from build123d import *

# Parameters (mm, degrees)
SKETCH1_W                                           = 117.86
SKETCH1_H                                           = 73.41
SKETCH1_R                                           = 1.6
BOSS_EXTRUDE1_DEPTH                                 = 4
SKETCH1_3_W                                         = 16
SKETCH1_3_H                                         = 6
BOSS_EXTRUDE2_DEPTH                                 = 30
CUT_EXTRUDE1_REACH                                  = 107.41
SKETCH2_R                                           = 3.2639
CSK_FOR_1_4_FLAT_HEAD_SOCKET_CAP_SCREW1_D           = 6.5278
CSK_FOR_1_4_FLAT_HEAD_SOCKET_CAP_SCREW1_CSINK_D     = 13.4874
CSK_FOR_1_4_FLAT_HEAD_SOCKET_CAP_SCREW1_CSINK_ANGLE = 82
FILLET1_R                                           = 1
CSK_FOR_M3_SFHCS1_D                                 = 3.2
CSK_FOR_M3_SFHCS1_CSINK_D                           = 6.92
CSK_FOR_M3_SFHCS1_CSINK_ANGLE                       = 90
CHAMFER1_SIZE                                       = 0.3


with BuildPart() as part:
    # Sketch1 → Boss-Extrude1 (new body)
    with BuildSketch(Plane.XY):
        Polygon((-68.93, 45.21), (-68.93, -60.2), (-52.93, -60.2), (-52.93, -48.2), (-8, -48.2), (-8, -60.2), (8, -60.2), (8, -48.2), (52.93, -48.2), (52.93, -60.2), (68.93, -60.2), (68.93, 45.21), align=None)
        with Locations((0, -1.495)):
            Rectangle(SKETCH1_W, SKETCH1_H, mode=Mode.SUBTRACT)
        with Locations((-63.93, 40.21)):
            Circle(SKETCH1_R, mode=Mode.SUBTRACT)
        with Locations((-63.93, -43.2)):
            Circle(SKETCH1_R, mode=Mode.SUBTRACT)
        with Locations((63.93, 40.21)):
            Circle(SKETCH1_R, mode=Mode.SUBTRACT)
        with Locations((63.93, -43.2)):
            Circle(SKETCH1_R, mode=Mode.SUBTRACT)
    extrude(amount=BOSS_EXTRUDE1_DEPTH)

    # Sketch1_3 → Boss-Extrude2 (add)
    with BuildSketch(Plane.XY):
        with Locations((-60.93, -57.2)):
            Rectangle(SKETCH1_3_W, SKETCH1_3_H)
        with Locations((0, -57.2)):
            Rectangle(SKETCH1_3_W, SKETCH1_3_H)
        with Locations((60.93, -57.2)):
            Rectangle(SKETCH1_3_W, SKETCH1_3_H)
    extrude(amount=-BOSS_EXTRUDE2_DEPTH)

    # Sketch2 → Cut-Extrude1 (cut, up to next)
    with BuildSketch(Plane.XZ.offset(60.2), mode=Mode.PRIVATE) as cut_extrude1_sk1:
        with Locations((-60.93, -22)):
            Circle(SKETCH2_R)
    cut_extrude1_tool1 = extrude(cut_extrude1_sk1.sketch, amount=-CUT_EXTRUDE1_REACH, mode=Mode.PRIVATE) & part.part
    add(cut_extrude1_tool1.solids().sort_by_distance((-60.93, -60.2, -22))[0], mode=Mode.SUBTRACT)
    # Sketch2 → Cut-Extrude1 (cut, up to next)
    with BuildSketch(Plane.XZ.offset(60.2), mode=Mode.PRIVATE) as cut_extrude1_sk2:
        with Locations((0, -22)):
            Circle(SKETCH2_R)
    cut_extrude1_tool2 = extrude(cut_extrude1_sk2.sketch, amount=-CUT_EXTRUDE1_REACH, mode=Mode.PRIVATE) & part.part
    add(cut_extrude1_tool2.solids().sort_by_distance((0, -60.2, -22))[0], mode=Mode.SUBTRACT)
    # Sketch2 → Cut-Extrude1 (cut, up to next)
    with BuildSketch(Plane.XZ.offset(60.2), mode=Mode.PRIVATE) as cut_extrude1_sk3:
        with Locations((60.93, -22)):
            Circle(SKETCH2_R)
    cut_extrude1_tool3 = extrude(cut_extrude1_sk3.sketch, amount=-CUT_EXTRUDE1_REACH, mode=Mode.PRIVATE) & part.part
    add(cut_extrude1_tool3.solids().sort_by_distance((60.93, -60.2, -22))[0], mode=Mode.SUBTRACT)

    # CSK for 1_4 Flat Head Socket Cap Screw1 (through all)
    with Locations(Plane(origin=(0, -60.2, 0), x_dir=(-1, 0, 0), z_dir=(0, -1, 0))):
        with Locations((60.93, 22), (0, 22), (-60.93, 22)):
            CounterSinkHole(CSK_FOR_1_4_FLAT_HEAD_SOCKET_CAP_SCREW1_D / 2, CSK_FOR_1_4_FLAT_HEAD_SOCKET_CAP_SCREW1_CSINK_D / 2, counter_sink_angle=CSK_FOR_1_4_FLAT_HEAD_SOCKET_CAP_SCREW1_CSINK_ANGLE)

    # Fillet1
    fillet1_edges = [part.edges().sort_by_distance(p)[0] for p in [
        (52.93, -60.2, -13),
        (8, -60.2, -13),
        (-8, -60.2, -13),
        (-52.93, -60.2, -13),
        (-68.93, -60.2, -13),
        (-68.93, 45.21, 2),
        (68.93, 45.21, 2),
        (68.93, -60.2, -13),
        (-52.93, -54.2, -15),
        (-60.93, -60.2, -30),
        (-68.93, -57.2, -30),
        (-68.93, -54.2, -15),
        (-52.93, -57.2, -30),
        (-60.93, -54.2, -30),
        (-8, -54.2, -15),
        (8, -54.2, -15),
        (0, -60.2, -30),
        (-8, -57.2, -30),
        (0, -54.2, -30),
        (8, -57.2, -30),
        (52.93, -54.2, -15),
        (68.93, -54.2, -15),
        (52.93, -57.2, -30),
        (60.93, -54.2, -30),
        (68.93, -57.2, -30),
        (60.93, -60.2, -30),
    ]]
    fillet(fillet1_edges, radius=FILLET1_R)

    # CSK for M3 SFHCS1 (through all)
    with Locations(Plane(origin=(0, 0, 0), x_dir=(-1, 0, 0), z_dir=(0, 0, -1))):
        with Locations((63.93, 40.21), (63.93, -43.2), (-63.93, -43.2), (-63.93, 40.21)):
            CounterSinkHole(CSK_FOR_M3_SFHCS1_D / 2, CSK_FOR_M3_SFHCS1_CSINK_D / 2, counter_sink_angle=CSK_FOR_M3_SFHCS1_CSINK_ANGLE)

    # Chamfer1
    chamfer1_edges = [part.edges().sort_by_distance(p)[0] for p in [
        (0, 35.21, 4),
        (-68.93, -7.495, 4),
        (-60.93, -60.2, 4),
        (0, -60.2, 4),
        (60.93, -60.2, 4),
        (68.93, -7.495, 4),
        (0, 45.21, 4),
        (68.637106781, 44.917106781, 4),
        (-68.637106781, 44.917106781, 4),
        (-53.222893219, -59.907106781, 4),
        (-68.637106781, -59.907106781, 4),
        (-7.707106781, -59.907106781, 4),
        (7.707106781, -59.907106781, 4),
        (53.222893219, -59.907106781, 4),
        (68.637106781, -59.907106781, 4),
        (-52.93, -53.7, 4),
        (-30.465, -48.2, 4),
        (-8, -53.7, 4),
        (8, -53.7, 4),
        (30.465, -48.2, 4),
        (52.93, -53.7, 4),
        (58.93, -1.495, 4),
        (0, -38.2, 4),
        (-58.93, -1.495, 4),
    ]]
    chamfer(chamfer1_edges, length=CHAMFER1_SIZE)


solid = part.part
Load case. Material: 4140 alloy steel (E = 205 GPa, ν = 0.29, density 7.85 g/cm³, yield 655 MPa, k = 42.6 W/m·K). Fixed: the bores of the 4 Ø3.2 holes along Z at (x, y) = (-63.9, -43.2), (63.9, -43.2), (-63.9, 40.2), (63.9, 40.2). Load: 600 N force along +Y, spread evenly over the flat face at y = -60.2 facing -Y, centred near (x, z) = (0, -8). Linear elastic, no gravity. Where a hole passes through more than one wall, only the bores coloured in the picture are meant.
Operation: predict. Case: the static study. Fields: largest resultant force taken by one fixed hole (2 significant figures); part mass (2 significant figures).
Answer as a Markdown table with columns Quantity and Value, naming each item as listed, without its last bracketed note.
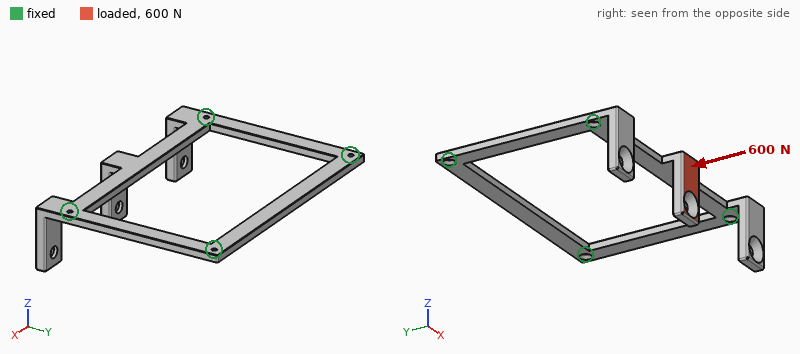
| Quantity | Value |
|---|---|
| largest resultant force taken by one fixed hole | 210 N |
| part mass | 210 g |
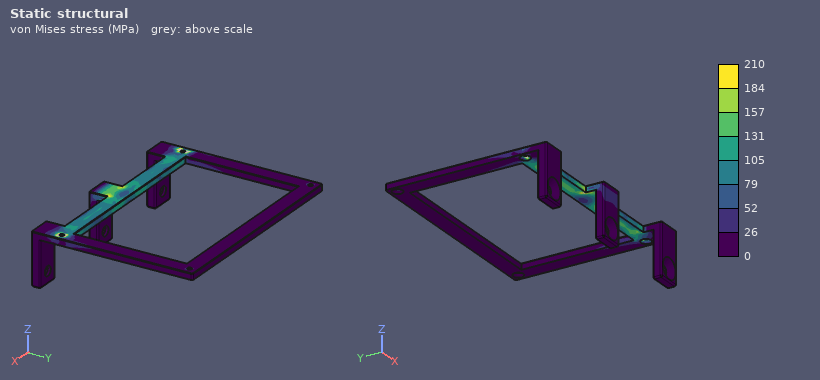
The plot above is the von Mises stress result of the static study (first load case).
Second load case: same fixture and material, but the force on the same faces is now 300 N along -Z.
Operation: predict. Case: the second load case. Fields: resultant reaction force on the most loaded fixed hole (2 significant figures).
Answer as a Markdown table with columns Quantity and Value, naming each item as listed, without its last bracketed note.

| Quantity | Value |
|---|---|
| resultant reaction force on the most loaded fixed hole | 220 N |
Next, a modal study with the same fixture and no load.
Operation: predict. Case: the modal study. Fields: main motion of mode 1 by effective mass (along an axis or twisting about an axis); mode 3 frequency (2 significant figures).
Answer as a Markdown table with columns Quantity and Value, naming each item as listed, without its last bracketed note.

| Quantity | Value |
|---|---|
| main motion of mode 1 by effective mass | along Z |
| mode 3 frequency | 1200 Hz |
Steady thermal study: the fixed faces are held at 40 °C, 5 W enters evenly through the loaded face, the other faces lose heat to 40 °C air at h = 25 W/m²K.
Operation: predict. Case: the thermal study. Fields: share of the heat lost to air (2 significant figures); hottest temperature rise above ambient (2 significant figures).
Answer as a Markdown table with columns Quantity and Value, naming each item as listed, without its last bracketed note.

| Quantity | Value |
|---|---|
| share of the heat lost to air | 70 % |
| hottest temperature rise above ambient | 54 K |
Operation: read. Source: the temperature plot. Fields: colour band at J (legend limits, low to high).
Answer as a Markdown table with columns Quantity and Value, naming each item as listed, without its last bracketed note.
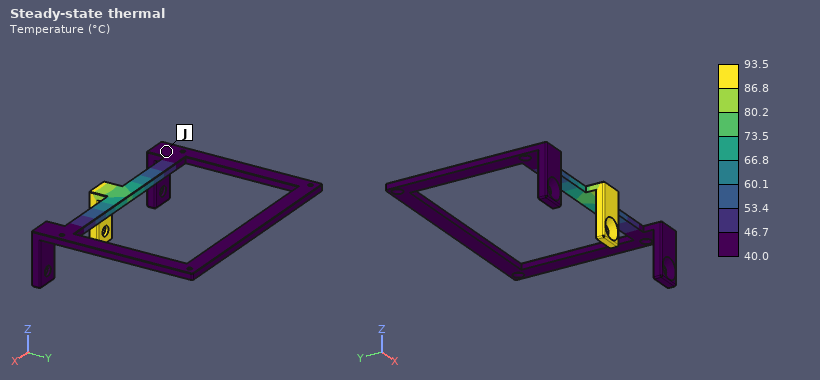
| Quantity | Value |
|---|---|
| colour band at J | 40.0 to 46.7 °C |
